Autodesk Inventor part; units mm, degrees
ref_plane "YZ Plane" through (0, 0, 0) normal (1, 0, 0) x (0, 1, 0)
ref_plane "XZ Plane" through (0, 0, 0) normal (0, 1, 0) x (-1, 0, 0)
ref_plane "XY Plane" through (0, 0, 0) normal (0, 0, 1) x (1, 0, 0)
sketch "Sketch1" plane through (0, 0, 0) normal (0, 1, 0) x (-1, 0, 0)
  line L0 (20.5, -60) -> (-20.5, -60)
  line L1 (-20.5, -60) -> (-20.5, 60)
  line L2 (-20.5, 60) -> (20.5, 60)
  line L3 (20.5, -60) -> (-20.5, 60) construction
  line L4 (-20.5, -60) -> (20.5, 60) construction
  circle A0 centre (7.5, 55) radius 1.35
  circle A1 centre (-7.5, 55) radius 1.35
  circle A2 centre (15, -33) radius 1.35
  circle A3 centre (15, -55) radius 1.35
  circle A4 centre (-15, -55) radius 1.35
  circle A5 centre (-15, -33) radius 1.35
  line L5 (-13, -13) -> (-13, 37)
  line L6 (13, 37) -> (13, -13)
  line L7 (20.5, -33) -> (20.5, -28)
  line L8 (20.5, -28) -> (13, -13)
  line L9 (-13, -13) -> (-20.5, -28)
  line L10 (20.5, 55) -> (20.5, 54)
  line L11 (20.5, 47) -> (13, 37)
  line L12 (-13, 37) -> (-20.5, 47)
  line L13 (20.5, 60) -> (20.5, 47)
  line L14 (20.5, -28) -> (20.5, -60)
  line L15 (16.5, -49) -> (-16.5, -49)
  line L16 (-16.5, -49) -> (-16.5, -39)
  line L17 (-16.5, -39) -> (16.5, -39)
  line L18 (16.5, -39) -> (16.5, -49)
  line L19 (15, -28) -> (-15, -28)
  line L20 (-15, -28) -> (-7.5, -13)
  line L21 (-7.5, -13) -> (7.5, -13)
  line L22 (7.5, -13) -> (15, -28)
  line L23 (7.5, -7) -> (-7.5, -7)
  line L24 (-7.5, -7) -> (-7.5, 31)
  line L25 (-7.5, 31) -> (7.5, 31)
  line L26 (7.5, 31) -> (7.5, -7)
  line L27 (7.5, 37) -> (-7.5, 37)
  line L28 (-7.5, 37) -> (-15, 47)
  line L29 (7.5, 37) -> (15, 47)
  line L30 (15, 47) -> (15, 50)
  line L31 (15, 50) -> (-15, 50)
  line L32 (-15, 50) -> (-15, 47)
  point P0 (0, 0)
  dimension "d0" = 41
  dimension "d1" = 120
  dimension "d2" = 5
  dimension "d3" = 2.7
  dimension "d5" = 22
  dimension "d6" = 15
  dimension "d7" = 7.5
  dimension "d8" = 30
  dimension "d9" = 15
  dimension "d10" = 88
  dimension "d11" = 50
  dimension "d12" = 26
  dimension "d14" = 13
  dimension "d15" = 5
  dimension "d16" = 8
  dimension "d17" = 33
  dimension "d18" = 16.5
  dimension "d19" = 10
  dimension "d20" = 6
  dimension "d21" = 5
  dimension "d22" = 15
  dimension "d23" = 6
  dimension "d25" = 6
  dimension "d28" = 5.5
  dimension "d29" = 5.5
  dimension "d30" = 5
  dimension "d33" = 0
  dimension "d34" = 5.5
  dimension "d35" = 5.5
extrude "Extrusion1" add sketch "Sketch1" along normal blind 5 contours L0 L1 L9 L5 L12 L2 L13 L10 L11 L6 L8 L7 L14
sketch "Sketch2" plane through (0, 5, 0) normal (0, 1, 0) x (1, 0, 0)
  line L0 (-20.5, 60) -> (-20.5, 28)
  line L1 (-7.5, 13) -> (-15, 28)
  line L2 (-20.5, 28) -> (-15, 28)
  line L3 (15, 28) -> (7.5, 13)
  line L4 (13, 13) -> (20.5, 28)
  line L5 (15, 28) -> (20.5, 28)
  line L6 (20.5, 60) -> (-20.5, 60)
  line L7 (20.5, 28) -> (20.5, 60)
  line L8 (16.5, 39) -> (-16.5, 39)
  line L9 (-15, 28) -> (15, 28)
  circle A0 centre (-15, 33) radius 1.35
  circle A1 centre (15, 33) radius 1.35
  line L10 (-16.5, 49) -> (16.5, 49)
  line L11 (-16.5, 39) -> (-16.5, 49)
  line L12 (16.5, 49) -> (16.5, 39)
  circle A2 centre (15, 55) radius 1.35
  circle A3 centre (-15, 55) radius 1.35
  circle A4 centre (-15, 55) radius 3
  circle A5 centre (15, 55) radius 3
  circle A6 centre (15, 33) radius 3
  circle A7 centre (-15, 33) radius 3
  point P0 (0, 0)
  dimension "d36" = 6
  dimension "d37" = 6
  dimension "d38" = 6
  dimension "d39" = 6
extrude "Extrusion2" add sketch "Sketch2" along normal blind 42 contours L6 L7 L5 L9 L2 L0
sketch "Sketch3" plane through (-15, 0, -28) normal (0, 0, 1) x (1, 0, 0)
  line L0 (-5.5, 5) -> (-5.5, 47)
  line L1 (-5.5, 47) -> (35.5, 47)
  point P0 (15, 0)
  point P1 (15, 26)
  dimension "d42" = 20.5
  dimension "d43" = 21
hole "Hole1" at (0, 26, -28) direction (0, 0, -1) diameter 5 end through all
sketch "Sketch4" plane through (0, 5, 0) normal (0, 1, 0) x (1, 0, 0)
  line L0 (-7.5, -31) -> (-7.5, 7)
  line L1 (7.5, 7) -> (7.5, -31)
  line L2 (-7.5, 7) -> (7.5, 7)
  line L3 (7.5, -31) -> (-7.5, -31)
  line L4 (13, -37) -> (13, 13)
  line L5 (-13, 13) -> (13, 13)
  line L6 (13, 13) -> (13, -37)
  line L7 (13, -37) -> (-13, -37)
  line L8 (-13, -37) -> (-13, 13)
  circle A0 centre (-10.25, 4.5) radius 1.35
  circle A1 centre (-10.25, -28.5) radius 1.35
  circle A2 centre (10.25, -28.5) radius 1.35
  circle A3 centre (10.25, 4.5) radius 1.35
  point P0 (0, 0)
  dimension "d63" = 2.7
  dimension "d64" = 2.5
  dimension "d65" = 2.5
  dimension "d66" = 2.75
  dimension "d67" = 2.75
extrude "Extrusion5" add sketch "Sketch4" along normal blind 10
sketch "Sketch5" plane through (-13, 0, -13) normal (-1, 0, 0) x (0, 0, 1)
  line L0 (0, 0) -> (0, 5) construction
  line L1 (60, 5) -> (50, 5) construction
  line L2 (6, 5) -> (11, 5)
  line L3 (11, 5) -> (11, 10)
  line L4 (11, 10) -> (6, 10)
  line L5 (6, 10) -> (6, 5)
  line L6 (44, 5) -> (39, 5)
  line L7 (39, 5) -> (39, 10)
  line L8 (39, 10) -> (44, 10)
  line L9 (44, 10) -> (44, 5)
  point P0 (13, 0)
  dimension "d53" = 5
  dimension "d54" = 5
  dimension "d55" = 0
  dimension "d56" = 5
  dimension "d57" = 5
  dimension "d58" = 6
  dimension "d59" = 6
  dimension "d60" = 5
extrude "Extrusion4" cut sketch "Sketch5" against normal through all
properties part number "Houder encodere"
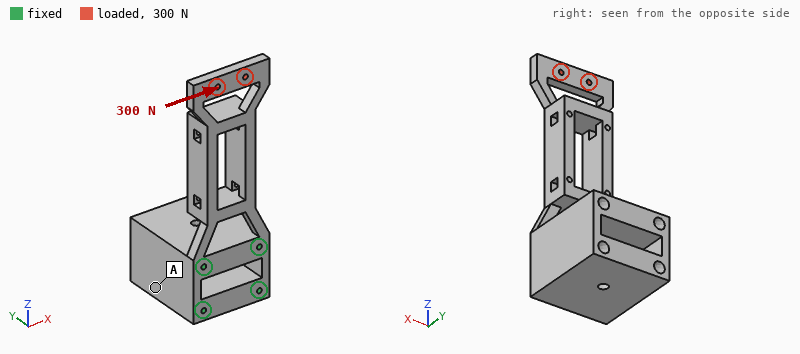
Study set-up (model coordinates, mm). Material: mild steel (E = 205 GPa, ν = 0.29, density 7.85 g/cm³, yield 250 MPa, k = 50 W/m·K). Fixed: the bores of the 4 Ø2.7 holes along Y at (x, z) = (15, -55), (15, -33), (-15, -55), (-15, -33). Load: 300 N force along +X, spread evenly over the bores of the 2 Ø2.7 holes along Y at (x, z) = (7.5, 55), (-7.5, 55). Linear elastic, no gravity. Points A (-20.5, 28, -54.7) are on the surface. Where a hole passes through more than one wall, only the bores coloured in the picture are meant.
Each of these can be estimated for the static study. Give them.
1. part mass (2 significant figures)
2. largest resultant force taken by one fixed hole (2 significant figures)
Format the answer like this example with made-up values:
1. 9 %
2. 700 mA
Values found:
1. 430 g
2. 770 N
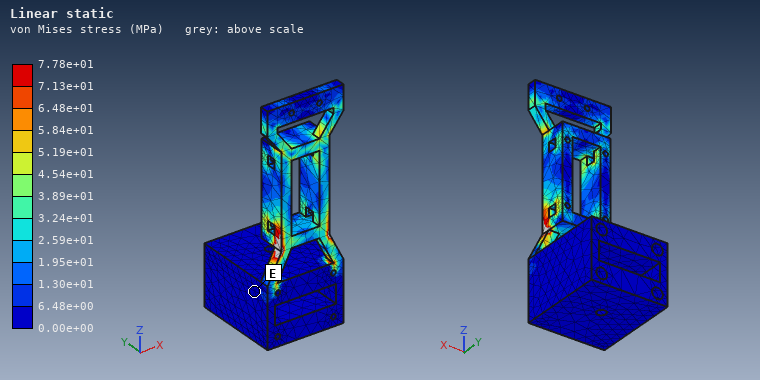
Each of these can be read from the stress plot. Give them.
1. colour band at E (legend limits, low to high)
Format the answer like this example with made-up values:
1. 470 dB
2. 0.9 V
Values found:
1. 0.00e+00 to 6.48e+00 MPa
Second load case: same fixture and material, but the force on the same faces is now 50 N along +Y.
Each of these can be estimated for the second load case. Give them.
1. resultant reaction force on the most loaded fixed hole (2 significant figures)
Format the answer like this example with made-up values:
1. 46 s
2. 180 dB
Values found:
1. 96 N
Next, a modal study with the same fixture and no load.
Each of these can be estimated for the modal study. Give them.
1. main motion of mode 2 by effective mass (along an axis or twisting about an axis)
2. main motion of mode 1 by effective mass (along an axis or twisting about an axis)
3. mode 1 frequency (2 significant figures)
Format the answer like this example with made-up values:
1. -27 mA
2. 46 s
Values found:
1. along X
2. along Y
3. 330 Hz
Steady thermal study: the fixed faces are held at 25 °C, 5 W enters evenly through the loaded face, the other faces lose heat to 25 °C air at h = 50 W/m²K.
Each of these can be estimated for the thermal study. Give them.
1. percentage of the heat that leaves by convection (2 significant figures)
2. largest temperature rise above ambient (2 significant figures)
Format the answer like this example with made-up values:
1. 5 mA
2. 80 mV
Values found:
1. 93 %
2. 39 K
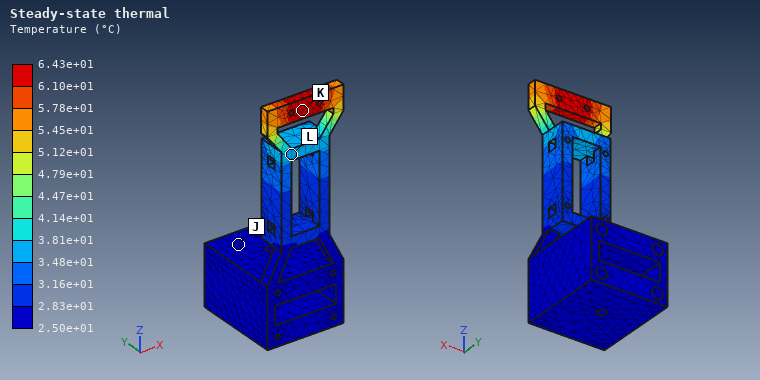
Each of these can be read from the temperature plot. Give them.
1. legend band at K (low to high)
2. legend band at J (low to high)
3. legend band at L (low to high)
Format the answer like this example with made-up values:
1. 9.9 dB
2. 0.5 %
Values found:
1. 6.10e+01 to 6.43e+01 °C
2. 2.50e+01 to 2.83e+01 °C
3. 3.48e+01 to 3.81e+01 °C
